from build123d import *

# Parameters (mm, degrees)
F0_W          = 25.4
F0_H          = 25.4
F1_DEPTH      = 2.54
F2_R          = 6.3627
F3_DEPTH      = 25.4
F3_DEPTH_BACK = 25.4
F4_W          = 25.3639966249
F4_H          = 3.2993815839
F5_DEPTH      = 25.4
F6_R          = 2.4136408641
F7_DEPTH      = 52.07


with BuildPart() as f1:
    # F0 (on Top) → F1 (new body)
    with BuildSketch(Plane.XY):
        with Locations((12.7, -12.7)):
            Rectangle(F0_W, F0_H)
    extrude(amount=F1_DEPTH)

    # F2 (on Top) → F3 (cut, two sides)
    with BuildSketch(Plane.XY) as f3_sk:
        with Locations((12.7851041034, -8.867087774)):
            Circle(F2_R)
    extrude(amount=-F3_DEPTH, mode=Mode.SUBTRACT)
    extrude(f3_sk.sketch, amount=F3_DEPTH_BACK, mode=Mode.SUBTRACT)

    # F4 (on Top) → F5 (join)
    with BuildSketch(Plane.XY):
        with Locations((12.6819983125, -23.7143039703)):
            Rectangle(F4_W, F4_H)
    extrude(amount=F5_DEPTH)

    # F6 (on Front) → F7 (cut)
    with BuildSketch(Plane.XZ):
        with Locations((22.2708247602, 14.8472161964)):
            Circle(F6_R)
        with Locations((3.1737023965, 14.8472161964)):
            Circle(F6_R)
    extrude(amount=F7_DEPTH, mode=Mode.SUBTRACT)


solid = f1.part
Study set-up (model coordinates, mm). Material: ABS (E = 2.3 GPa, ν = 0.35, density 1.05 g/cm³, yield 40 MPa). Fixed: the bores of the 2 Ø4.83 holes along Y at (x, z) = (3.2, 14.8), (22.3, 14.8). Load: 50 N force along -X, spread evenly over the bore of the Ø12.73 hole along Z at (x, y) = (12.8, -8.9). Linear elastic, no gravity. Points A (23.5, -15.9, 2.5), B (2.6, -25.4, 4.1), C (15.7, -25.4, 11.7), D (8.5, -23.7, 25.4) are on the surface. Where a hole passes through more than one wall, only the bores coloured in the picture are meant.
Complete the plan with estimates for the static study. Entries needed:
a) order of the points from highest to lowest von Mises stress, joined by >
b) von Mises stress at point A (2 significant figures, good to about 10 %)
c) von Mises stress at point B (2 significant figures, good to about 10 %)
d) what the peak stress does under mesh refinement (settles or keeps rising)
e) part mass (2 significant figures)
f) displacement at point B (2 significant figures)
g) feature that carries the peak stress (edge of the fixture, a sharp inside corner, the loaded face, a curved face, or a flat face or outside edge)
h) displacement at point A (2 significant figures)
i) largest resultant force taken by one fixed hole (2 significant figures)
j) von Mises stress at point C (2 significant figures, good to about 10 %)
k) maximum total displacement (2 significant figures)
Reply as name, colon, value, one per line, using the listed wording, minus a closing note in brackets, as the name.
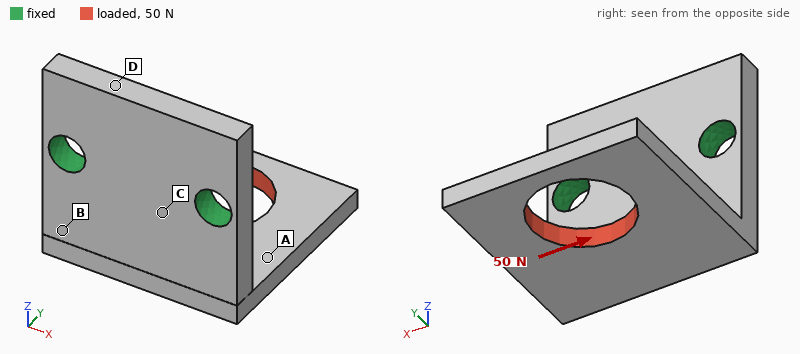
order of the points from highest to lowest von Mises stress, joined by >: B > A > C > D
von Mises stress at point A: 4.5 MPa
von Mises stress at point B: 6.7 MPa
what the peak stress does under mesh refinement: keeps rising
part mass: 3.3 g
displacement at point B: 0.11 mm
feature that carries the peak stress: edge of the fixture
displacement at point A: 0.23 mm
largest resultant force taken by one fixed hole: 55 N
von Mises stress at point C: 3.0 MPa
maximum total displacement: 0.52 mm
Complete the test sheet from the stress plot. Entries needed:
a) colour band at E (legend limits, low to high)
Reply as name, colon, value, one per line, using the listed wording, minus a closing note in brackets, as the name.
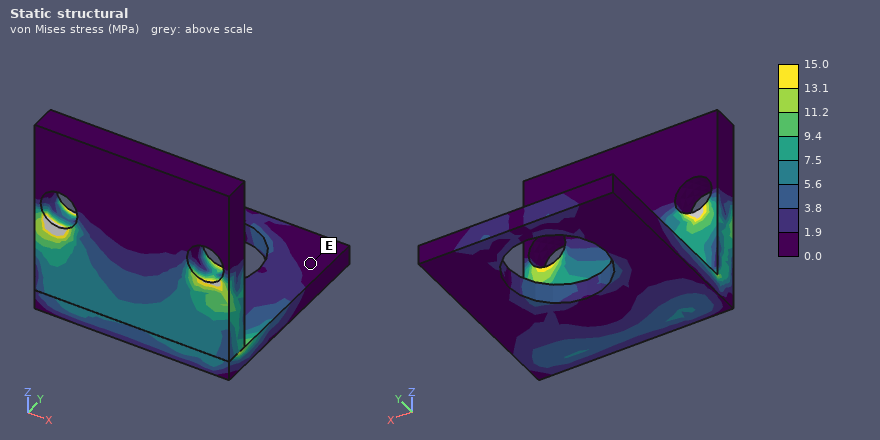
colour band at E: 0.0 to 1.9 MPa
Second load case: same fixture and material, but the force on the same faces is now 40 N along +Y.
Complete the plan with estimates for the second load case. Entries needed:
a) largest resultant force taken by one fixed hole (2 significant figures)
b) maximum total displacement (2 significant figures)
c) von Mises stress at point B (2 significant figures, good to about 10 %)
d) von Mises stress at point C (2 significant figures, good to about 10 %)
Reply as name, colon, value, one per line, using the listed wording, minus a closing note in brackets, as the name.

largest resultant force taken by one fixed hole: 20 N
maximum total displacement: 0.45 mm
von Mises stress at point B: 2.6 MPa
von Mises stress at point C: 5.0 MPa
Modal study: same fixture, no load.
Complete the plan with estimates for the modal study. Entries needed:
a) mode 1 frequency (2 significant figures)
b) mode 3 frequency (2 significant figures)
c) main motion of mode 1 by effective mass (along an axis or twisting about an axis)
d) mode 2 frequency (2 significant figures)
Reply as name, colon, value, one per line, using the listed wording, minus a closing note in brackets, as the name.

mode 1 frequency: 870 Hz
mode 3 frequency: 2200 Hz
main motion of mode 1 by effective mass: along Z
mode 2 frequency: 1700 Hz
